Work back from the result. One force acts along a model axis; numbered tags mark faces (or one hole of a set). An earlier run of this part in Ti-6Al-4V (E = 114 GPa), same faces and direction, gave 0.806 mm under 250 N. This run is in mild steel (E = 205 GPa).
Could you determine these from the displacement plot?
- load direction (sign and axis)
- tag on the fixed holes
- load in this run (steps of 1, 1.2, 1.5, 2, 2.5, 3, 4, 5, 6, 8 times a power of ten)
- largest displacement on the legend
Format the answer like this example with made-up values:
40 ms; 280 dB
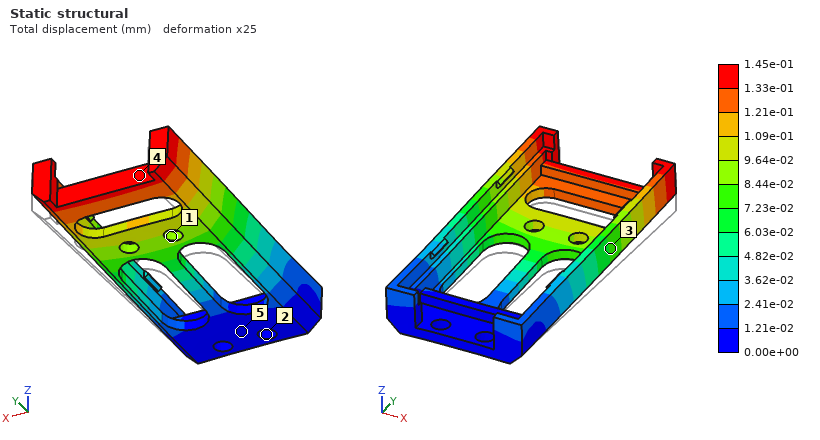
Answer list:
+Z; 2; 80 N; 1.45e-01 mm
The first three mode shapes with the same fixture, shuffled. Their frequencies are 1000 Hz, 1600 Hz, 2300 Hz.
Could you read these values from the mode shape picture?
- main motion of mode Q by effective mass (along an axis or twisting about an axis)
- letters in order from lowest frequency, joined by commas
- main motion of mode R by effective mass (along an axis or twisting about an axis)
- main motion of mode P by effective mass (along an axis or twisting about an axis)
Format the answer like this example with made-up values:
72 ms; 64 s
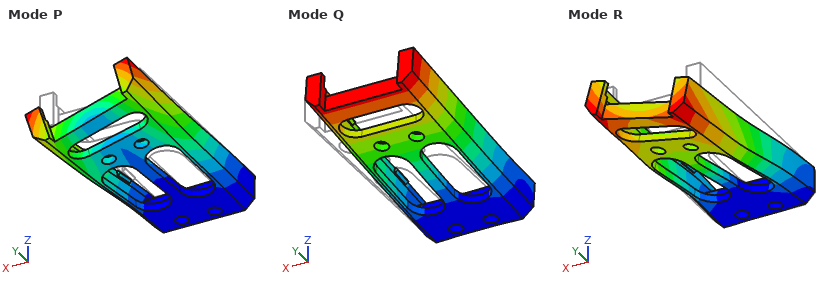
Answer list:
along Z; Q, P, R; along X; along X
